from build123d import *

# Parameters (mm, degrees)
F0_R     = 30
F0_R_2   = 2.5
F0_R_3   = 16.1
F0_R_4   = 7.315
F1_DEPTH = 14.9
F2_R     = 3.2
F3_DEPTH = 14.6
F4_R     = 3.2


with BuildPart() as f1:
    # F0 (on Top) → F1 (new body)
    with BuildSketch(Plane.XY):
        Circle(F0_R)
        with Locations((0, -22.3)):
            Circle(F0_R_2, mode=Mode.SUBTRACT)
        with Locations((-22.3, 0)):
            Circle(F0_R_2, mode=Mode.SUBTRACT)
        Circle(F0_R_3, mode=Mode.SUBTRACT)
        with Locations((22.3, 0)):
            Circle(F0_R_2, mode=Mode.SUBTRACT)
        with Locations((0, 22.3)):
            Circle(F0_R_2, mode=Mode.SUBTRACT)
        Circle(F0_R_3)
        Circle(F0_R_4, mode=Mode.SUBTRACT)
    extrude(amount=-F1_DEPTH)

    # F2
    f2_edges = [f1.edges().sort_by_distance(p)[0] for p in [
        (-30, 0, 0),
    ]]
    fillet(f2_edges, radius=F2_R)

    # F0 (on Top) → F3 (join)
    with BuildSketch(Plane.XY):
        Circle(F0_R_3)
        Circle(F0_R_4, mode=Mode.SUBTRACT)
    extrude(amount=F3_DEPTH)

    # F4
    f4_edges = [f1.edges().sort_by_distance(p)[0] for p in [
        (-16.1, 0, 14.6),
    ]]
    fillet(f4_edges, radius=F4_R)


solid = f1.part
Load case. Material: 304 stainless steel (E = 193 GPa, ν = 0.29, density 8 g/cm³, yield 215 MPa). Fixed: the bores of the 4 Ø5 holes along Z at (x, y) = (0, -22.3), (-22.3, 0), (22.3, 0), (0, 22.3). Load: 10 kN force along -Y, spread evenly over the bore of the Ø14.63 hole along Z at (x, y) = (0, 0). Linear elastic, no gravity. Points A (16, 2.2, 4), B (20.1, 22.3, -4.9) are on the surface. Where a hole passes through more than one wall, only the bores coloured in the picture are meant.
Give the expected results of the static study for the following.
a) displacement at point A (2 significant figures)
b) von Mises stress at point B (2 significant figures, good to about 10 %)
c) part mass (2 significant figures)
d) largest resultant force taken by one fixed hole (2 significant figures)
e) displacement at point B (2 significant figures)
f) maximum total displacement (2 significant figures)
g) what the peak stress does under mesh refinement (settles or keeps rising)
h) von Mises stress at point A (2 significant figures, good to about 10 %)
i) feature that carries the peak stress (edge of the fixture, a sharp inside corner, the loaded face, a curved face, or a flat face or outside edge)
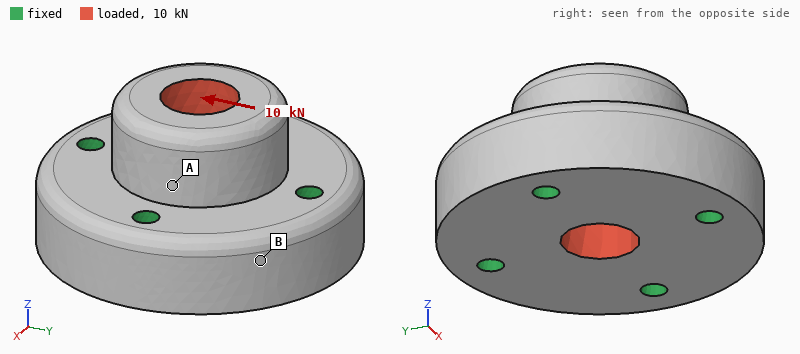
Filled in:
1.6 µm
4.4 MPa
380 g
3.5 kN
0.72 µm
3.6 µm
keeps rising
11 MPa
a sharp inside corner
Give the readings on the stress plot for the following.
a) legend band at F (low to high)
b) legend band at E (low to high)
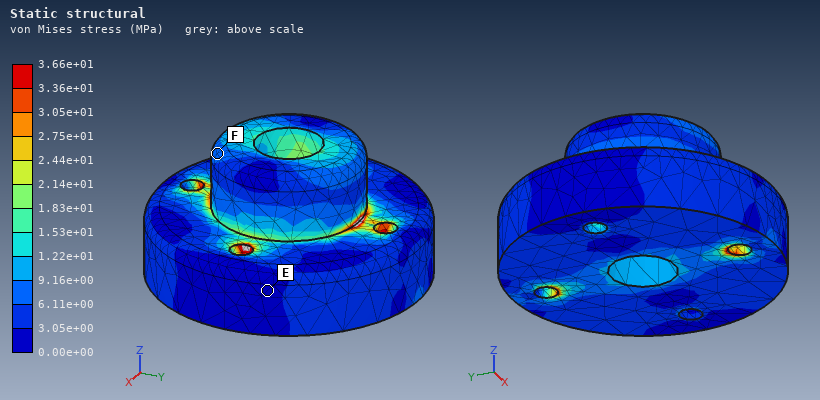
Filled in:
6.11e+00 to 9.16e+00 MPa
0.00e+00 to 3.05e+00 MPa
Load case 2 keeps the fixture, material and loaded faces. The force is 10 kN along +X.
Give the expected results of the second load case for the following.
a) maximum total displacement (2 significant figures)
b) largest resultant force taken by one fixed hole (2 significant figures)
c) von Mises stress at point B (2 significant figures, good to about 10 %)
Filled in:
3.6 µm
3.5 kN
4.2 MPa
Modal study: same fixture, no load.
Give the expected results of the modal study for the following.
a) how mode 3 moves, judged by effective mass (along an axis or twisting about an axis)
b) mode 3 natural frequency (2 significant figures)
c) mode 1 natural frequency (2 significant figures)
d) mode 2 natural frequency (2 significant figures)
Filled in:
along Z
28 kHz
25 kHz
25 kHz
